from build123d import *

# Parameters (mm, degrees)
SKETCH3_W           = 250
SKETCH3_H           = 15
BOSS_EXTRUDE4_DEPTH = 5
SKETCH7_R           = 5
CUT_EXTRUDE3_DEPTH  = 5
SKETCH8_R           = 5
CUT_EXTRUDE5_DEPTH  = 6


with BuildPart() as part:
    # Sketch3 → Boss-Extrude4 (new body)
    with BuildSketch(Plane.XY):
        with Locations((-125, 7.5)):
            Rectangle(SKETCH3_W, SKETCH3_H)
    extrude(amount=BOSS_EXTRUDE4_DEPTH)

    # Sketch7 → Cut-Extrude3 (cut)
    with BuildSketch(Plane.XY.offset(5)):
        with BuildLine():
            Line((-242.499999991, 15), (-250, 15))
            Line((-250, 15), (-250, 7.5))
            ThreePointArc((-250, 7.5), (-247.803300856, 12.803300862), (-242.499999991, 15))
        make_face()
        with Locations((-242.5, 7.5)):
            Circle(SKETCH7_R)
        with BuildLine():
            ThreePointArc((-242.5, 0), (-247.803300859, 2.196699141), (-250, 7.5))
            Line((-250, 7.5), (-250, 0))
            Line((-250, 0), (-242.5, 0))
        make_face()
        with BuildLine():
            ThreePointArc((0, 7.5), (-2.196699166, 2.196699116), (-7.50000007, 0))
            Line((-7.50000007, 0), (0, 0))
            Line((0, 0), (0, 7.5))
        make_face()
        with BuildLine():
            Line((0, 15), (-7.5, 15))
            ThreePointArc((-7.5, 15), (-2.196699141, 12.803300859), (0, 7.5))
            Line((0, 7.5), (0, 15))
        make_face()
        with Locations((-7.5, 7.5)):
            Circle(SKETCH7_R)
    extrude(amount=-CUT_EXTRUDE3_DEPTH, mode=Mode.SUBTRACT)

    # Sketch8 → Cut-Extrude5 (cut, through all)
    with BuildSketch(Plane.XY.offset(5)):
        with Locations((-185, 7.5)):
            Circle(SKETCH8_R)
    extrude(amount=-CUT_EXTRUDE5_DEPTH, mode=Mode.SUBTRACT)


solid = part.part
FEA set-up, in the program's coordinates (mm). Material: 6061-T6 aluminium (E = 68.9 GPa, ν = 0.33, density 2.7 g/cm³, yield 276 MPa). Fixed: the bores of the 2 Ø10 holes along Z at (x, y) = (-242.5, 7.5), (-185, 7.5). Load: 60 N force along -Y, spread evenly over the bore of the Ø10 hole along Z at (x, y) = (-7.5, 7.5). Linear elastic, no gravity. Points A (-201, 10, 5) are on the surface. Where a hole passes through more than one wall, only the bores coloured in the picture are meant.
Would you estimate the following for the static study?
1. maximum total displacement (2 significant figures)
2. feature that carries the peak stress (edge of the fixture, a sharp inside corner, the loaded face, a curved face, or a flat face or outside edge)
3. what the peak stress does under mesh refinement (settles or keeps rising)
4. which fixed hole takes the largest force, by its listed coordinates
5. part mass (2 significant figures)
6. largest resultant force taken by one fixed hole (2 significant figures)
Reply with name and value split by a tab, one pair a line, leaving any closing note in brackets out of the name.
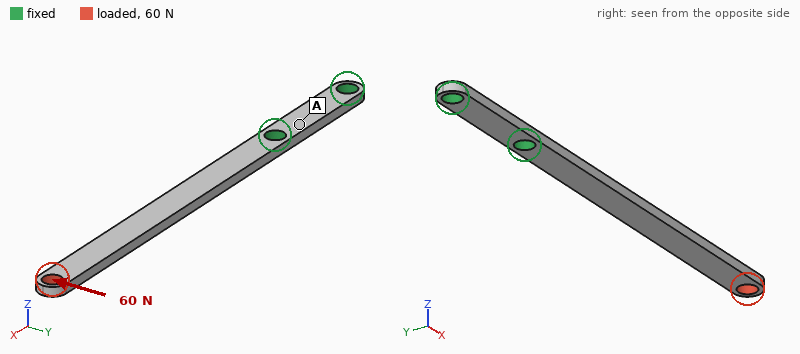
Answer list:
maximum total displacement	1.2 mm
feature that carries the peak stress	edge of the fixture
what the peak stress does under mesh refinement	keeps rising
which fixed hole takes the largest force, by its listed coordinates	(-185, 7.5)
part mass	47 g
largest resultant force taken by one fixed hole	66 N
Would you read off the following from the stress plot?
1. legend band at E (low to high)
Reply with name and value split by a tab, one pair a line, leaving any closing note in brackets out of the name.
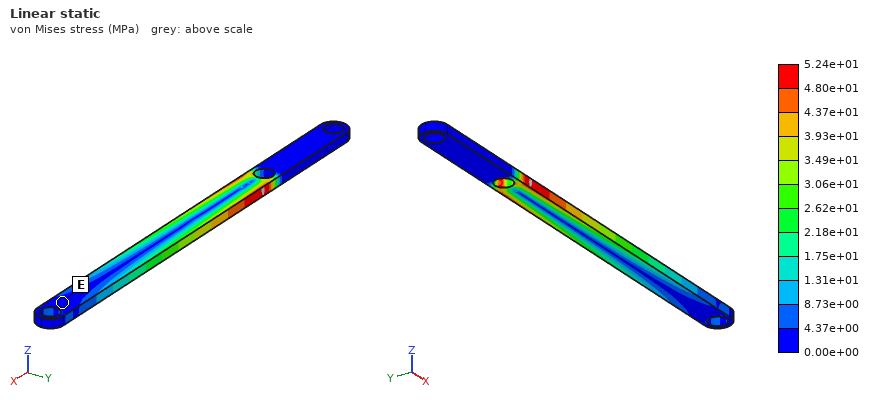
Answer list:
legend band at E	0.00e+00 to 4.37e+00 MPa
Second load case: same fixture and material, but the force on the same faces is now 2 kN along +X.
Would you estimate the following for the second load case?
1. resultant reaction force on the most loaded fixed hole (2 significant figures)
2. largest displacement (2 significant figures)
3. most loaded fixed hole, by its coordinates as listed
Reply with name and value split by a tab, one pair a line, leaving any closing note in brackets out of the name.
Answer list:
resultant reaction force on the most loaded fixed hole	2.0 kN
largest displacement	85 µm
most loaded fixed hole, by its coordinates as listed	(-185, 7.5)
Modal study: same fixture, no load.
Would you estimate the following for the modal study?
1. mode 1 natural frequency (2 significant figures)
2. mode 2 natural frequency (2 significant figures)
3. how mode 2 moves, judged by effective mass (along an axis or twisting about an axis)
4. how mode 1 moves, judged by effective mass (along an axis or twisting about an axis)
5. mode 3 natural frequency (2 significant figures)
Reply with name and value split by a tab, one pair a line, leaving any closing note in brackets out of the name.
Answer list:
mode 1 natural frequency	130 Hz
mode 2 natural frequency	390 Hz
how mode 2 moves, judged by effective mass	along Y
how mode 1 moves, judged by effective mass	along Z
mode 3 natural frequency	830 Hz
